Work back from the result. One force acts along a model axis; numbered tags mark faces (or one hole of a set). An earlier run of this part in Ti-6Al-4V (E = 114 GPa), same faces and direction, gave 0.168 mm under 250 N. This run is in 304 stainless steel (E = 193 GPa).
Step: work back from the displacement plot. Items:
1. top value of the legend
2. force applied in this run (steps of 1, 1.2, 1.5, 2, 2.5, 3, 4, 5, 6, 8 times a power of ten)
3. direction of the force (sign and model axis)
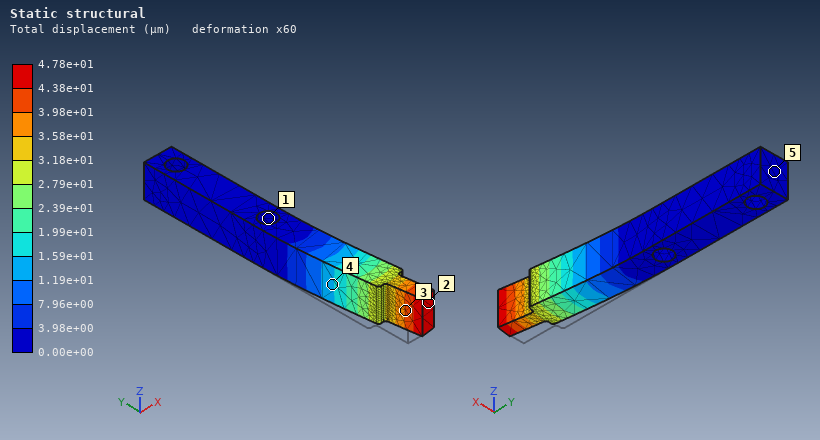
4.78e+01 µm
120 N
+X
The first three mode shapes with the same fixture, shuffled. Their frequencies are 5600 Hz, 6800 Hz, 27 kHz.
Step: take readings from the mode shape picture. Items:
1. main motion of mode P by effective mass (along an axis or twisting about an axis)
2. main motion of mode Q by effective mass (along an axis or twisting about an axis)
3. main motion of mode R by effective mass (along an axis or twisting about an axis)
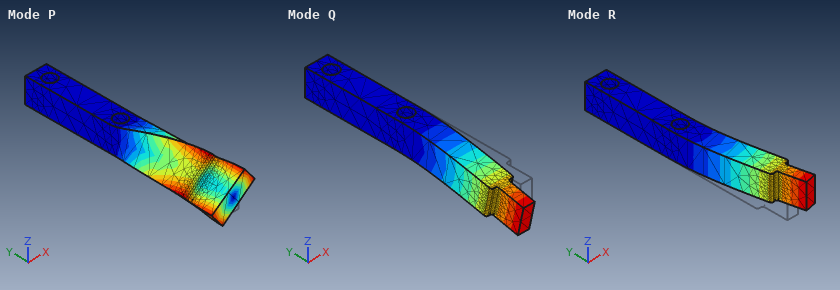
twisting about Y
along Z
along X
